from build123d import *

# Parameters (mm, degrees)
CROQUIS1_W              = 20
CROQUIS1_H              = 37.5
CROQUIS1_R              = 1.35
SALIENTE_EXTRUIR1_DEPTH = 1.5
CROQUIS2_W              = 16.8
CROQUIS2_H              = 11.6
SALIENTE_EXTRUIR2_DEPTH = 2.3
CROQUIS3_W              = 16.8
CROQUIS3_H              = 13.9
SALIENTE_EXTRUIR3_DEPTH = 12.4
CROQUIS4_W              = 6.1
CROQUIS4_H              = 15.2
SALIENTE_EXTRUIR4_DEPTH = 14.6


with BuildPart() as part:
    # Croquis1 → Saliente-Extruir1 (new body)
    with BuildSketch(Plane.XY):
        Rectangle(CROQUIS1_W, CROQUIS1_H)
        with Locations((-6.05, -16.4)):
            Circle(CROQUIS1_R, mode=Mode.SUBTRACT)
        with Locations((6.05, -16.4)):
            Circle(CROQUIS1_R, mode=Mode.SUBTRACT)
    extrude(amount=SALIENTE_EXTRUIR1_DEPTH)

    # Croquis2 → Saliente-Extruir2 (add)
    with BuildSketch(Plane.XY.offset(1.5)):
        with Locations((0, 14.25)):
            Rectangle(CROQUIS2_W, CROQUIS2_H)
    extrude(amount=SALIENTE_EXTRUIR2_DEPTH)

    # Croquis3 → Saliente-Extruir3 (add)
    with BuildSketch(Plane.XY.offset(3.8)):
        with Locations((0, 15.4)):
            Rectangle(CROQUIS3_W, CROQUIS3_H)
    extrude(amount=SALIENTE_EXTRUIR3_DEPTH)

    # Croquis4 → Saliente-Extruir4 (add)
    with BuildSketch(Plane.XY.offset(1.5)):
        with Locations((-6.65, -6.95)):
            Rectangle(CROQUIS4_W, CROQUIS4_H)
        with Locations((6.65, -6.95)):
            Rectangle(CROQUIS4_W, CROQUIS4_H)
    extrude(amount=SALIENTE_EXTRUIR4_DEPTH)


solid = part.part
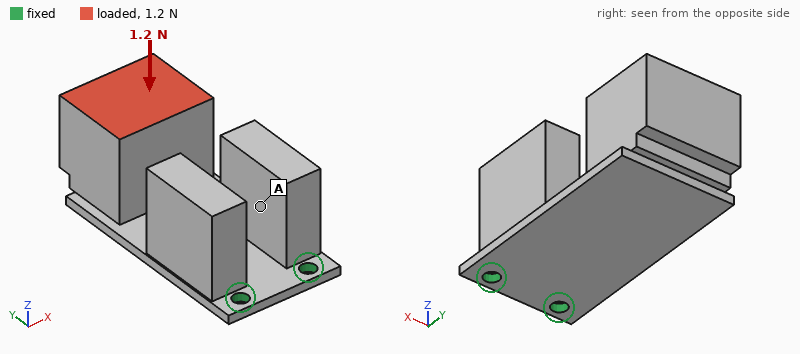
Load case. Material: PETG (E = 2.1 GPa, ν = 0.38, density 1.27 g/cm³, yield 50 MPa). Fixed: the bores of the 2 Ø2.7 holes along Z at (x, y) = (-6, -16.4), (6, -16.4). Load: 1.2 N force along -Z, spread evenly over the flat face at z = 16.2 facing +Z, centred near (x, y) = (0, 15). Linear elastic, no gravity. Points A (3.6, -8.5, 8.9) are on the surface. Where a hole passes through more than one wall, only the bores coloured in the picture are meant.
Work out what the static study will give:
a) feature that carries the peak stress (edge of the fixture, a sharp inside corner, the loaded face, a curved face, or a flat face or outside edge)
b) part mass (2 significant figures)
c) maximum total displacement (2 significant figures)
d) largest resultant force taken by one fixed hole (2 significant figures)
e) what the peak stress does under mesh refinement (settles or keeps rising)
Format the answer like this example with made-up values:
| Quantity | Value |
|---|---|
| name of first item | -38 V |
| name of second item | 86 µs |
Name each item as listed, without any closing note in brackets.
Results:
| Quantity | Value |
|---|---|
| feature that carries the peak stress | edge of the fixture |
| part mass | 9.1 g |
| maximum total displacement | 0.50 mm |
| largest resultant force taken by one fixed hole | 0.77 N |
| what the peak stress does under mesh refinement | keeps rising |
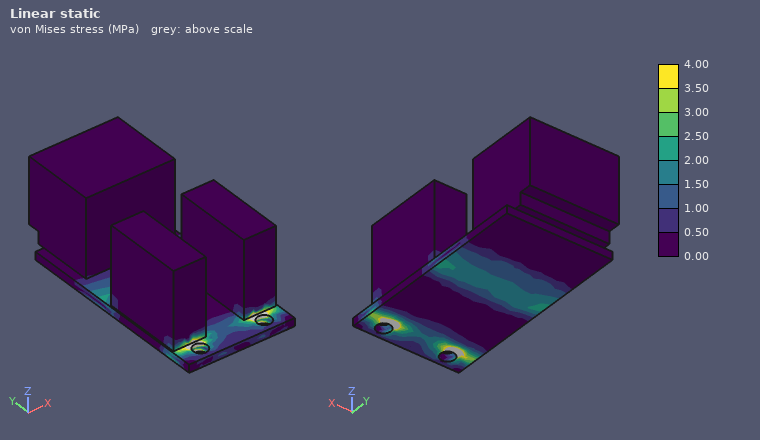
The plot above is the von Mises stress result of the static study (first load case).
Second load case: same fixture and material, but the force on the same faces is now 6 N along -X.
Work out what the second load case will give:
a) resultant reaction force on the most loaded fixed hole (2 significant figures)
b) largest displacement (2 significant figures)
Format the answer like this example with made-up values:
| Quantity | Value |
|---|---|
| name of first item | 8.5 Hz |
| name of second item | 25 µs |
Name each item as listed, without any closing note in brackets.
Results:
| Quantity | Value |
|---|---|
| resultant reaction force on the most loaded fixed hole | 14 N |
| largest displacement | 0.52 mm |
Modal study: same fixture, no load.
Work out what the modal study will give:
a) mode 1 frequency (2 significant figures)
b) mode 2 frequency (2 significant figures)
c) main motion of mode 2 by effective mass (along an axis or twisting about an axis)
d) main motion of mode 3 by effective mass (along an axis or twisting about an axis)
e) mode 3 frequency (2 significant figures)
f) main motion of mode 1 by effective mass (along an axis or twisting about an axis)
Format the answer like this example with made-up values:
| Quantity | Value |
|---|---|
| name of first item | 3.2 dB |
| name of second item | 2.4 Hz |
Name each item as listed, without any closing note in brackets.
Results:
| Quantity | Value |
|---|---|
| mode 1 frequency | 130 Hz |
| mode 2 frequency | 390 Hz |
| main motion of mode 2 by effective mass | along X |
| main motion of mode 3 by effective mass | along Z |
| mode 3 frequency | 450 Hz |
| main motion of mode 1 by effective mass | along Z |
